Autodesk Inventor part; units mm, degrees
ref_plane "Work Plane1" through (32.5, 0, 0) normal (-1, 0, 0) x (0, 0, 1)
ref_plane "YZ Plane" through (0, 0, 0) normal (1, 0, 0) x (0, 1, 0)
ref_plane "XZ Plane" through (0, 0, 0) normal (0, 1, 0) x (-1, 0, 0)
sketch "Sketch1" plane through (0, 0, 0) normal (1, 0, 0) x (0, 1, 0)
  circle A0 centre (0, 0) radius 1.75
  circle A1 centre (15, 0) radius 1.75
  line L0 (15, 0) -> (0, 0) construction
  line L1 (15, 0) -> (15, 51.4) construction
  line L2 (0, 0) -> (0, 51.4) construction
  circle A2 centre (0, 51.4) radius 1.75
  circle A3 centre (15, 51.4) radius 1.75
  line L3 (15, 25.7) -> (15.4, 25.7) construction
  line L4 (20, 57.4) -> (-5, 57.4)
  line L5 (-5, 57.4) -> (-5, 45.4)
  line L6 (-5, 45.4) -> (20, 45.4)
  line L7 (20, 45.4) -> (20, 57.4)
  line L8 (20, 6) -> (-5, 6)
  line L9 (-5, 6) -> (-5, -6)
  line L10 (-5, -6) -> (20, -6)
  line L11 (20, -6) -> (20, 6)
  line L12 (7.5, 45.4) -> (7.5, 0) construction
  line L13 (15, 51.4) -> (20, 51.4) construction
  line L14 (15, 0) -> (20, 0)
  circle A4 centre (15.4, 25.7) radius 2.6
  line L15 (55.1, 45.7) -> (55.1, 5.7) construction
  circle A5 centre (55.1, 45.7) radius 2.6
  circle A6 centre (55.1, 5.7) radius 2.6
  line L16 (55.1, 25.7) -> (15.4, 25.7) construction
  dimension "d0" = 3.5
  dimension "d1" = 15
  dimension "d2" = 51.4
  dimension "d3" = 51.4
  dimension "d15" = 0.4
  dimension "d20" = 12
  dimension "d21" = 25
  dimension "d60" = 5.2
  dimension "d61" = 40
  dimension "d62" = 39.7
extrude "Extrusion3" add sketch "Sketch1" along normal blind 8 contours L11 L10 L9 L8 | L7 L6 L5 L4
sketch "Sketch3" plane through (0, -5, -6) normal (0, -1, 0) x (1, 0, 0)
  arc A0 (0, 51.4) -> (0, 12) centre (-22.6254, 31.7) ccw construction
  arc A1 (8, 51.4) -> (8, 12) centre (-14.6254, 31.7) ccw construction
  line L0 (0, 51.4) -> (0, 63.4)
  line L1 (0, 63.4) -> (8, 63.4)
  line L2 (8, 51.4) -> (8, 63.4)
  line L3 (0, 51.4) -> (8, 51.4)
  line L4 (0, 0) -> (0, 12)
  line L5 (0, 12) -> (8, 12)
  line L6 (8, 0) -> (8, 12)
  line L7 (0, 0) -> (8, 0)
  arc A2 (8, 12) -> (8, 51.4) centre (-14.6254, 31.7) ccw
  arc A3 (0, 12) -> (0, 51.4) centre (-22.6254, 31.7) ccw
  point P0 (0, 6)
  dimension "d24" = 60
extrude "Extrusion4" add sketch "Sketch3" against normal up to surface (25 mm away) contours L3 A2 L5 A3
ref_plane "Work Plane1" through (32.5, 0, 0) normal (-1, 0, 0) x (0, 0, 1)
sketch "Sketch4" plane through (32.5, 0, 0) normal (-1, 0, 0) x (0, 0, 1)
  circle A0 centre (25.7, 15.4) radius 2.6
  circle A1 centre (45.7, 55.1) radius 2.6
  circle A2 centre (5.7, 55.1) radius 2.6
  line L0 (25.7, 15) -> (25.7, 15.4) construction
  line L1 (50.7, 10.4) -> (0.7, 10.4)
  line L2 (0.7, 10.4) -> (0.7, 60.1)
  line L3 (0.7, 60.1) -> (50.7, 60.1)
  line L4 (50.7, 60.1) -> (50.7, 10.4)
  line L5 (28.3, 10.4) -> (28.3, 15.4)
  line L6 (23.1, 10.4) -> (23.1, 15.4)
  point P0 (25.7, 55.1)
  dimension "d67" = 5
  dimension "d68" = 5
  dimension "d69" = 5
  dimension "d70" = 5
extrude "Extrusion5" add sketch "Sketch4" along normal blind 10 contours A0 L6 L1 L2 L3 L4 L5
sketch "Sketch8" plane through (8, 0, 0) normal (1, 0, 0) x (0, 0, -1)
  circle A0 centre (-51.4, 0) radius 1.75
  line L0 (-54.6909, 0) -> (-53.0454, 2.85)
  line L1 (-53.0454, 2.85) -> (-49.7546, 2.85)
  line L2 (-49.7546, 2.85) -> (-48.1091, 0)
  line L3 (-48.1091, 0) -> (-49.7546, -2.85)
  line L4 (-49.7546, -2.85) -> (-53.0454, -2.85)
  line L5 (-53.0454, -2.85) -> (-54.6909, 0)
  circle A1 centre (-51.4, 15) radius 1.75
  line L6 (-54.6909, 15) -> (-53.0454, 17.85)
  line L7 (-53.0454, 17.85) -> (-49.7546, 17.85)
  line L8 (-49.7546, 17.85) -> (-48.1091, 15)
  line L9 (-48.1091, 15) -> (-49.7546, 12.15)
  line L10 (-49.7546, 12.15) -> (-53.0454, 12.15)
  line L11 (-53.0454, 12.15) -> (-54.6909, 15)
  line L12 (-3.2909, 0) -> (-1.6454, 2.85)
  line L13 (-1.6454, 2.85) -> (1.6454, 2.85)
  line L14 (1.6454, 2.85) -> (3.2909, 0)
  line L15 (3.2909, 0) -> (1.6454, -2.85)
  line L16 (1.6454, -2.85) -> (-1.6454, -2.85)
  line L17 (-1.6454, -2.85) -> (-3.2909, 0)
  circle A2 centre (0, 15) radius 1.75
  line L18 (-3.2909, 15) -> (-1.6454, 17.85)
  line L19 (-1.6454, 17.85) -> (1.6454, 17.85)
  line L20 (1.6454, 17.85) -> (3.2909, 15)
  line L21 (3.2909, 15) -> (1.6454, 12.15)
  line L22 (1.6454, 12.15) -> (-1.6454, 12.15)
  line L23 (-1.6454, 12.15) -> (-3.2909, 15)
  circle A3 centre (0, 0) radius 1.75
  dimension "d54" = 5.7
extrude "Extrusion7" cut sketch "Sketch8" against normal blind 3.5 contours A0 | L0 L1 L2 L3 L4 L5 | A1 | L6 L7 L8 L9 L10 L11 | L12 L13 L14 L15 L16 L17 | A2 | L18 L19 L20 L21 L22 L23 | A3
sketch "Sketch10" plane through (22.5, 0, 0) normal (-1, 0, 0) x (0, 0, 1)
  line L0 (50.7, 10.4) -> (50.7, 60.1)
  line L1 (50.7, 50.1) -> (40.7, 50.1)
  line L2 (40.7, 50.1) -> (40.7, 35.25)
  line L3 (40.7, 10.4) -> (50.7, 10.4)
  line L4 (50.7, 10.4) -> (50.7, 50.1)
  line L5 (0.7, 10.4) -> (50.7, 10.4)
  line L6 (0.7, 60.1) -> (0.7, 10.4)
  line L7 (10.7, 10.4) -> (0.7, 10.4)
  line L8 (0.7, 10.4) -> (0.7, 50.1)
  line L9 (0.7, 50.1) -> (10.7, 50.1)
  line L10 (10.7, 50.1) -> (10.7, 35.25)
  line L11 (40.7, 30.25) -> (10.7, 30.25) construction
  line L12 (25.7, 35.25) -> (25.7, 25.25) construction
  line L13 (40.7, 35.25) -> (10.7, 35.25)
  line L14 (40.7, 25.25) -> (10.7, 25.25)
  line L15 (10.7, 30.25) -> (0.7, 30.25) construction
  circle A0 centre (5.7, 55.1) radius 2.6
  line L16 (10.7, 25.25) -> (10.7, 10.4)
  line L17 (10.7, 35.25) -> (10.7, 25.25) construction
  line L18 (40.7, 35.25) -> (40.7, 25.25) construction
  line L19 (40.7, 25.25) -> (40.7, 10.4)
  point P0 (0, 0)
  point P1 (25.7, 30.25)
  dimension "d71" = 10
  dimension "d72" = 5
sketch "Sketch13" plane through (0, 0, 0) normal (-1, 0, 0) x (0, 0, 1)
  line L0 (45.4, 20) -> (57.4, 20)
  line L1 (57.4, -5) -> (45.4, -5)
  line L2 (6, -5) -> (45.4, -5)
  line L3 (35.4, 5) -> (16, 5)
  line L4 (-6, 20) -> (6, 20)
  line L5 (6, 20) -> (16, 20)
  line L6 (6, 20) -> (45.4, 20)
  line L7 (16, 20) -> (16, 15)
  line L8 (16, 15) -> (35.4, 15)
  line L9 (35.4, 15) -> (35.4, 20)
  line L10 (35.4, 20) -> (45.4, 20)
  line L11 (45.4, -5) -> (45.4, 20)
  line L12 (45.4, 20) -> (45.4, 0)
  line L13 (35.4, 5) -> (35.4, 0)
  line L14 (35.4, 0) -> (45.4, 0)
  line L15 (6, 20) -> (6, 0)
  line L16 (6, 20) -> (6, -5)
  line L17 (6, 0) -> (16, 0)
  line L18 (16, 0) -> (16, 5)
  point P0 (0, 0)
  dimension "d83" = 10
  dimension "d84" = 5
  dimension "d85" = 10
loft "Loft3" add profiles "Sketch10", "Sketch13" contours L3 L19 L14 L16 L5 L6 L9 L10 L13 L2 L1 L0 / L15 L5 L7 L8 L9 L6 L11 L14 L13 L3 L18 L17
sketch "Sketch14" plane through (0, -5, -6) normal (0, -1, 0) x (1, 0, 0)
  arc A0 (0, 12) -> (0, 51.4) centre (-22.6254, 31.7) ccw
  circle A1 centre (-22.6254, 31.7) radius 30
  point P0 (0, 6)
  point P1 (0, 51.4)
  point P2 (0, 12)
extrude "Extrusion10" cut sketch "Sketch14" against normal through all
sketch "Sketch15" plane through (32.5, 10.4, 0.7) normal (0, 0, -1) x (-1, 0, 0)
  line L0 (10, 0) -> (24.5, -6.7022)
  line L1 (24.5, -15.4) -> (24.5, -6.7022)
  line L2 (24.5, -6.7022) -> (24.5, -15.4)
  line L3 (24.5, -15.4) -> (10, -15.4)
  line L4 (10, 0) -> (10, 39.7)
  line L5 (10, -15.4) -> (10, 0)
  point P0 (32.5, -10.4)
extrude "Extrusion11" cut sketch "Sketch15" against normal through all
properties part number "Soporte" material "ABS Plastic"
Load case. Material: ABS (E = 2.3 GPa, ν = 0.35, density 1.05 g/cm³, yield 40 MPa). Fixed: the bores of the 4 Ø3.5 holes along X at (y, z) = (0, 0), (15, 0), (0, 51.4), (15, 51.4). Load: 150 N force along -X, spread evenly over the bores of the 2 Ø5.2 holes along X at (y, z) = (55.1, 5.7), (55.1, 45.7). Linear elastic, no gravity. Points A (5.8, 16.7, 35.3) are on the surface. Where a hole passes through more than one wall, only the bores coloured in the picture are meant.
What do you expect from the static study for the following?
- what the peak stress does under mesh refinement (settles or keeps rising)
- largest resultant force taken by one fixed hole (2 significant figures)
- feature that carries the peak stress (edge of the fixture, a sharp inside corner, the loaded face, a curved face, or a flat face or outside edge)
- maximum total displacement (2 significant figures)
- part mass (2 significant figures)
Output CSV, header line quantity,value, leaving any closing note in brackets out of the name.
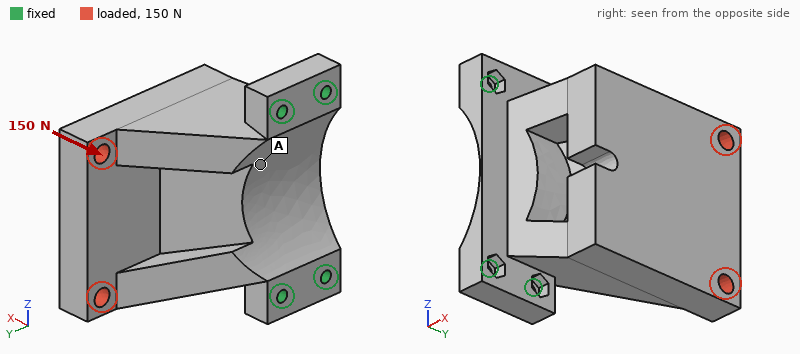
quantity,value
what the peak stress does under mesh refinement,keeps rising
largest resultant force taken by one fixed hole,280 N
feature that carries the peak stress,edge of the fixture
maximum total displacement,0.64 mm
part mass,49 g
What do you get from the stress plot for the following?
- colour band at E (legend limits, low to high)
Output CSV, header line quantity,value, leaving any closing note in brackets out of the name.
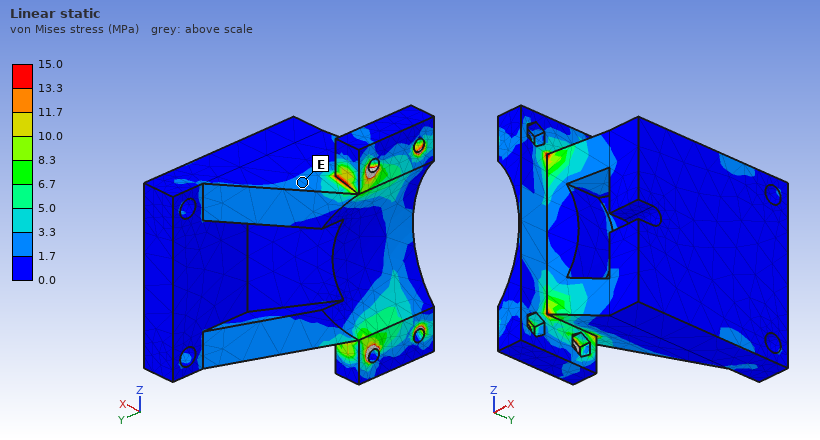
quantity,value
colour band at E,1.7 to 3.3 MPa
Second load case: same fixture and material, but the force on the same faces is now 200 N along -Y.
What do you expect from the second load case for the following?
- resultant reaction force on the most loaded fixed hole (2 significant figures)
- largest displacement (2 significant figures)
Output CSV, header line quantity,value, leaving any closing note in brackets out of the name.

quantity,value
resultant reaction force on the most loaded fixed hole,200 N
largest displacement,0.40 mm
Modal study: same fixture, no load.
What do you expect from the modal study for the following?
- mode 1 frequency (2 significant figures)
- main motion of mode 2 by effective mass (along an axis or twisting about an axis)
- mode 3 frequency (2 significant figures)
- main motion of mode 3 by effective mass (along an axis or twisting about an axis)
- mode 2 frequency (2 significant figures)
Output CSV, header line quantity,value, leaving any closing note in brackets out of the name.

quantity,value
mode 1 frequency,650 Hz
main motion of mode 2 by effective mass,along Z
mode 3 frequency,2100 Hz
main motion of mode 3 by effective mass,along Z
mode 2 frequency,1600 Hz
